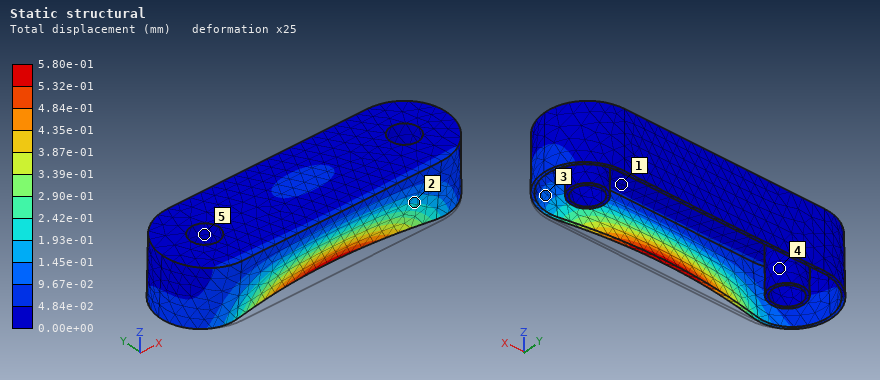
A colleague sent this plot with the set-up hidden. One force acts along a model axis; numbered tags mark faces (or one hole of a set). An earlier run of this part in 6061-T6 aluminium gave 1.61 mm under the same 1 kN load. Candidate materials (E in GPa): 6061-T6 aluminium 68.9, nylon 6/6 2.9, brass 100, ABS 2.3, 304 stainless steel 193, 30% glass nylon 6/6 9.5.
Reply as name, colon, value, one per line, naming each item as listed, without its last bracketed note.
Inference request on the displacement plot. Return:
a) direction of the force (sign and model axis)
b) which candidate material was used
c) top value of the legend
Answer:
direction of the force: +Y
which candidate material was used: 304 stainless steel
top value of the legend: 5.80e-01 mm
